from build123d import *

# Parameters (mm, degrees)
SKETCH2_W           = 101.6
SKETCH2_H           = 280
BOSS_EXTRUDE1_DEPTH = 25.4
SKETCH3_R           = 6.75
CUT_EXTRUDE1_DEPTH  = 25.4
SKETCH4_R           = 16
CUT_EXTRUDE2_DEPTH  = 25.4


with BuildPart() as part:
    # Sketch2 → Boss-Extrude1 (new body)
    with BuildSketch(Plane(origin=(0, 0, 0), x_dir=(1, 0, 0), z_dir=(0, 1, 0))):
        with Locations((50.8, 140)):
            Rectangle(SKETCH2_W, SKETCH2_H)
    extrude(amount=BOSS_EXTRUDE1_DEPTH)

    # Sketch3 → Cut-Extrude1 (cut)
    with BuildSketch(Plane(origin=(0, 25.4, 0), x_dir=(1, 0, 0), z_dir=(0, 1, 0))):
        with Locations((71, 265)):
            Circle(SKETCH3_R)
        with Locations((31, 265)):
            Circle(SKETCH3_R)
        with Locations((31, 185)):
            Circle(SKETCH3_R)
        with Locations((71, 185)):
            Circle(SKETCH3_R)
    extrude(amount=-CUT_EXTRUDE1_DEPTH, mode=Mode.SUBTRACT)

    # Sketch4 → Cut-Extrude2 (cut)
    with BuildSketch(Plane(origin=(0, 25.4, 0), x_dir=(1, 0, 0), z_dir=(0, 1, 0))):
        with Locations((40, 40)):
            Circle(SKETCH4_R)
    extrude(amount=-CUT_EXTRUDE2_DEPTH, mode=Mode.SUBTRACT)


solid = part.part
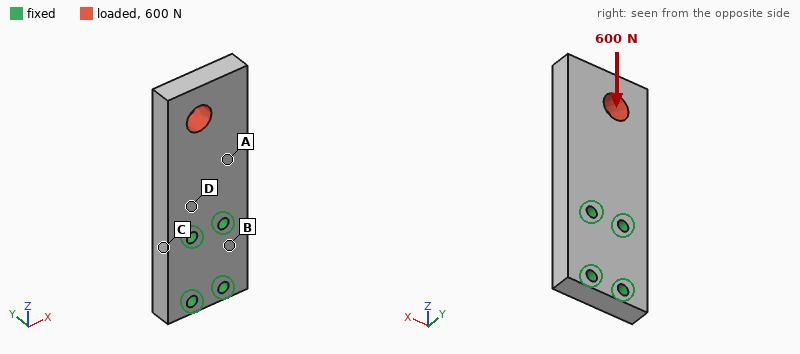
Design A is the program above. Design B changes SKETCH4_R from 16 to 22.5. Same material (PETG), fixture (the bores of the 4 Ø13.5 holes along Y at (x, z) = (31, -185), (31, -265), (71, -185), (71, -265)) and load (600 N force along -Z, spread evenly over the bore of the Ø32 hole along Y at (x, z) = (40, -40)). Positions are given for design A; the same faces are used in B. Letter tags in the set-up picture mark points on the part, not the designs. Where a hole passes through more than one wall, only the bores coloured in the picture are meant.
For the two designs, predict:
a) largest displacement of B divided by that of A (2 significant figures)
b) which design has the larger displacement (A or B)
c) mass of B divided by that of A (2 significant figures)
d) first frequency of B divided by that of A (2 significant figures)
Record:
1.2
B
0.97
1.0
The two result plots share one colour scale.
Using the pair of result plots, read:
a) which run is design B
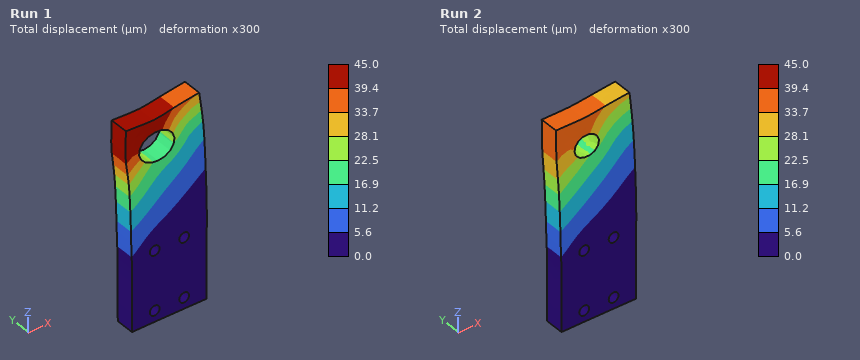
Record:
Run 1
